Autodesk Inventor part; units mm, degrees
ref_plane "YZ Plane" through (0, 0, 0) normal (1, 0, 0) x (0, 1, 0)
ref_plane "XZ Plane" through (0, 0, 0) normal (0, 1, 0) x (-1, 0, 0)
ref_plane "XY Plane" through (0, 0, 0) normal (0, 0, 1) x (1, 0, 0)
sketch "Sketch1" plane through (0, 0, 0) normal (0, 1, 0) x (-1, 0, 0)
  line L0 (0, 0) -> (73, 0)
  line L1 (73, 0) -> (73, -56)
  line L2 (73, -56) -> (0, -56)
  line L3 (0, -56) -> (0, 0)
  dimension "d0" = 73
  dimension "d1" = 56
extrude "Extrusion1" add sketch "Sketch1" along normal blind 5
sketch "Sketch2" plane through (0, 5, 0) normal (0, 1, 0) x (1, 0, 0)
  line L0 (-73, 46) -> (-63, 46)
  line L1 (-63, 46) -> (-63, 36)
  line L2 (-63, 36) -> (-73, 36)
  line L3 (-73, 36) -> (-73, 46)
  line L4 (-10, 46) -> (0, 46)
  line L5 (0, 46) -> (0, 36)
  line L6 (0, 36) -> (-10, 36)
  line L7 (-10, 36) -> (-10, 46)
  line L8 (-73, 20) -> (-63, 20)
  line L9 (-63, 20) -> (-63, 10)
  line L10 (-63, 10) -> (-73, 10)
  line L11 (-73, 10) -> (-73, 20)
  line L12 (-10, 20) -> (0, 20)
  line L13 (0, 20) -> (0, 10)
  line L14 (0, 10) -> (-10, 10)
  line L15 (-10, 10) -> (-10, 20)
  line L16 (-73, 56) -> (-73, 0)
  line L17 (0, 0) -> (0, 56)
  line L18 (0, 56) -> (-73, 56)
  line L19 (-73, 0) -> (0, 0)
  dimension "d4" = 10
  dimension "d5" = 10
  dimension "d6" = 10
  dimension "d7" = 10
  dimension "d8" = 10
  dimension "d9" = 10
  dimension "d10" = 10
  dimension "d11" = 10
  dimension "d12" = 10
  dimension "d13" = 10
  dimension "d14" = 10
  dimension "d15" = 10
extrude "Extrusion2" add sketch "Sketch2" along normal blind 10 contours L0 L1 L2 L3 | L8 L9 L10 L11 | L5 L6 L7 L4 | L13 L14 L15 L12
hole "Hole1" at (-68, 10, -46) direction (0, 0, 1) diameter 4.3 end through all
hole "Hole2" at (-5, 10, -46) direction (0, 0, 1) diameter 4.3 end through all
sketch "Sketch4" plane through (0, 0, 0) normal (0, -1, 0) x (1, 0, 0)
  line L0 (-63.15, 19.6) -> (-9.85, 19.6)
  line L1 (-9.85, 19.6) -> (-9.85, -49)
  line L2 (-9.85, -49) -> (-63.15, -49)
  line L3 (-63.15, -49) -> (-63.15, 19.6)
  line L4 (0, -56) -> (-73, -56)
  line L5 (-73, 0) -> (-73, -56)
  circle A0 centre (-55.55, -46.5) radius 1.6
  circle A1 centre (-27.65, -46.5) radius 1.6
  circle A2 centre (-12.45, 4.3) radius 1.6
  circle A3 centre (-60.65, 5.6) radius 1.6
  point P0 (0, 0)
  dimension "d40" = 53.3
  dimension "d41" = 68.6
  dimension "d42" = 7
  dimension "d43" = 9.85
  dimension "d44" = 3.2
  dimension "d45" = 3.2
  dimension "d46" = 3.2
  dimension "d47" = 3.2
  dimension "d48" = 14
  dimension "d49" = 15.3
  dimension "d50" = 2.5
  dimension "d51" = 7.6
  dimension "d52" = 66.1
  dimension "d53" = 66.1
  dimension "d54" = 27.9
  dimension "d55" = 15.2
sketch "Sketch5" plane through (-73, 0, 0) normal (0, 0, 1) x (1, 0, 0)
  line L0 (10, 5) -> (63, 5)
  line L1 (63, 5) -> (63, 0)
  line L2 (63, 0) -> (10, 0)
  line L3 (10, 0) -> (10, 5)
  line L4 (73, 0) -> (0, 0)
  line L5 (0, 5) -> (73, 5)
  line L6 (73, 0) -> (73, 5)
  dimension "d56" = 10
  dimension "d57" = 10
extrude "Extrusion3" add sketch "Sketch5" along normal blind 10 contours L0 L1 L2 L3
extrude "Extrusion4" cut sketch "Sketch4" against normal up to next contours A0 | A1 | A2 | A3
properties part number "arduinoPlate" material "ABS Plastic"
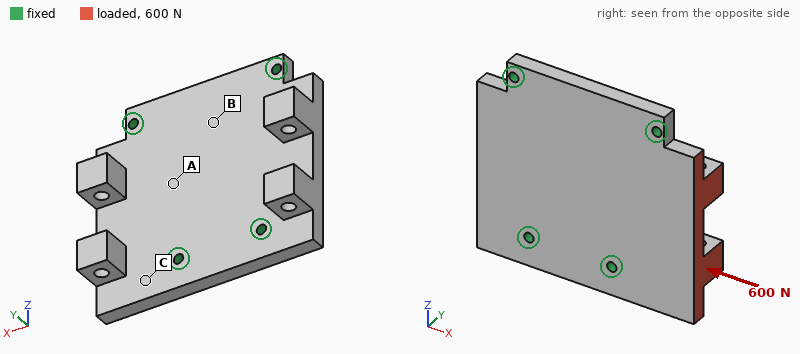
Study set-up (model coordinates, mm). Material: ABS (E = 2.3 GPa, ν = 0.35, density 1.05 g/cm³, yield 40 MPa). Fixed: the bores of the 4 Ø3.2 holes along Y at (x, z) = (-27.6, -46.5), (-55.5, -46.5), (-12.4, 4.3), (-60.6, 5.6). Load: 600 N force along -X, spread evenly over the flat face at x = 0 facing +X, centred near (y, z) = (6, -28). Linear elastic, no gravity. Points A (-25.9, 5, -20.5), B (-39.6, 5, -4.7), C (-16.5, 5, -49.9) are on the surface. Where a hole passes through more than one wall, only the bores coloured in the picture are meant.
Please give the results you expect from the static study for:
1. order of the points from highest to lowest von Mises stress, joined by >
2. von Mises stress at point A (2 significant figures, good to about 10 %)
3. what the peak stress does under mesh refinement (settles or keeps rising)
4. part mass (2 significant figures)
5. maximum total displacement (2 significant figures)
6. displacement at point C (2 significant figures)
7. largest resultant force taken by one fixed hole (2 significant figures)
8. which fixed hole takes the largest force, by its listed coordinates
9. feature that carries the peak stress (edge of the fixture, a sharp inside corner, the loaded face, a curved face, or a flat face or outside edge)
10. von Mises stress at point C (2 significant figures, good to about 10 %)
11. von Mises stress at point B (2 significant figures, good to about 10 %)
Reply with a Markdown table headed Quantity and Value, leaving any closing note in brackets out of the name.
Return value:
| Quantity | Value |
|---|---|
| order of the points from highest to lowest von Mises stress, joined by > | C > A > B |
| von Mises stress at point A | 5.2 MPa |
| what the peak stress does under mesh refinement | keeps rising |
| part mass | 28 g |
| maximum total displacement | 0.66 mm |
| displacement at point C | 0.11 mm |
| largest resultant force taken by one fixed hole | 280 N |
| which fixed hole takes the largest force, by its listed coordinates | (-27.6, -46.5) |
| feature that carries the peak stress | edge of the fixture |
| von Mises stress at point C | 9.4 MPa |
| von Mises stress at point B | 2.1 MPa |
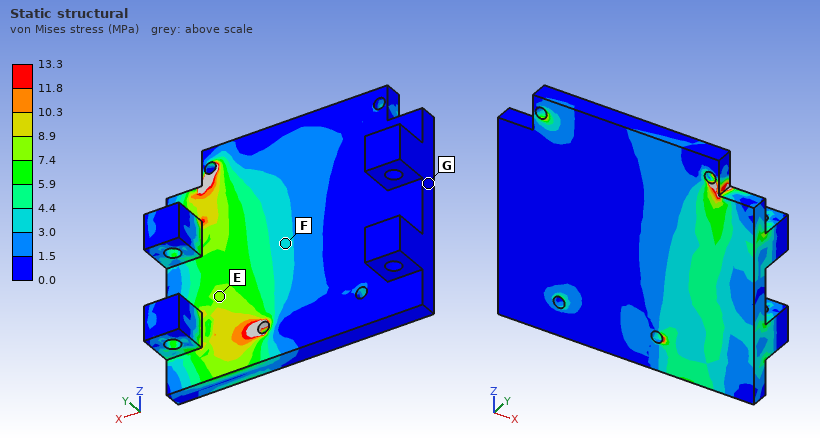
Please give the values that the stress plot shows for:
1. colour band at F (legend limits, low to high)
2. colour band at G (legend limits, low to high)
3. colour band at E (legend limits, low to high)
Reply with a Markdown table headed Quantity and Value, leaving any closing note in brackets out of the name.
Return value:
| Quantity | Value |
|---|---|
| colour band at F | 3.0 to 4.4 MPa |
| colour band at G | 0.0 to 1.5 MPa |
| colour band at E | 7.4 to 8.9 MPa |
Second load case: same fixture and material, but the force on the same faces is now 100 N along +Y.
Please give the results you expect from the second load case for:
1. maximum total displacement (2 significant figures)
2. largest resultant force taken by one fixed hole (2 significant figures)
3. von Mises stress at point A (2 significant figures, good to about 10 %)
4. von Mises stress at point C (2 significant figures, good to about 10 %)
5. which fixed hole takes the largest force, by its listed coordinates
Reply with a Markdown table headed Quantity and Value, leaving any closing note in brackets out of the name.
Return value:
| Quantity | Value |
|---|---|
| maximum total displacement | 0.66 mm |
| largest resultant force taken by one fixed hole | 76 N |
| von Mises stress at point A | 4.1 MPa |
| von Mises stress at point C | 6.1 MPa |
| which fixed hole takes the largest force, by its listed coordinates | (-27.6, -46.5) |
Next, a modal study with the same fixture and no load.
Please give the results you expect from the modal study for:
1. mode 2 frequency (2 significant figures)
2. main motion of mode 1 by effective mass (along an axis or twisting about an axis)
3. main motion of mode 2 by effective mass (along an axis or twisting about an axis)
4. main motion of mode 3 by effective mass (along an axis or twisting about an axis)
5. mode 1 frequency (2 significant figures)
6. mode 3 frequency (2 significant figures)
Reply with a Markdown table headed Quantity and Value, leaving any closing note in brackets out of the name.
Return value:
| Quantity | Value |
|---|---|
| mode 2 frequency | 1700 Hz |
| main motion of mode 1 by effective mass | along Y |
| main motion of mode 2 by effective mass | along Y |
| main motion of mode 3 by effective mass | along Y |
| mode 1 frequency | 1200 Hz |
| mode 3 frequency | 2100 Hz |
